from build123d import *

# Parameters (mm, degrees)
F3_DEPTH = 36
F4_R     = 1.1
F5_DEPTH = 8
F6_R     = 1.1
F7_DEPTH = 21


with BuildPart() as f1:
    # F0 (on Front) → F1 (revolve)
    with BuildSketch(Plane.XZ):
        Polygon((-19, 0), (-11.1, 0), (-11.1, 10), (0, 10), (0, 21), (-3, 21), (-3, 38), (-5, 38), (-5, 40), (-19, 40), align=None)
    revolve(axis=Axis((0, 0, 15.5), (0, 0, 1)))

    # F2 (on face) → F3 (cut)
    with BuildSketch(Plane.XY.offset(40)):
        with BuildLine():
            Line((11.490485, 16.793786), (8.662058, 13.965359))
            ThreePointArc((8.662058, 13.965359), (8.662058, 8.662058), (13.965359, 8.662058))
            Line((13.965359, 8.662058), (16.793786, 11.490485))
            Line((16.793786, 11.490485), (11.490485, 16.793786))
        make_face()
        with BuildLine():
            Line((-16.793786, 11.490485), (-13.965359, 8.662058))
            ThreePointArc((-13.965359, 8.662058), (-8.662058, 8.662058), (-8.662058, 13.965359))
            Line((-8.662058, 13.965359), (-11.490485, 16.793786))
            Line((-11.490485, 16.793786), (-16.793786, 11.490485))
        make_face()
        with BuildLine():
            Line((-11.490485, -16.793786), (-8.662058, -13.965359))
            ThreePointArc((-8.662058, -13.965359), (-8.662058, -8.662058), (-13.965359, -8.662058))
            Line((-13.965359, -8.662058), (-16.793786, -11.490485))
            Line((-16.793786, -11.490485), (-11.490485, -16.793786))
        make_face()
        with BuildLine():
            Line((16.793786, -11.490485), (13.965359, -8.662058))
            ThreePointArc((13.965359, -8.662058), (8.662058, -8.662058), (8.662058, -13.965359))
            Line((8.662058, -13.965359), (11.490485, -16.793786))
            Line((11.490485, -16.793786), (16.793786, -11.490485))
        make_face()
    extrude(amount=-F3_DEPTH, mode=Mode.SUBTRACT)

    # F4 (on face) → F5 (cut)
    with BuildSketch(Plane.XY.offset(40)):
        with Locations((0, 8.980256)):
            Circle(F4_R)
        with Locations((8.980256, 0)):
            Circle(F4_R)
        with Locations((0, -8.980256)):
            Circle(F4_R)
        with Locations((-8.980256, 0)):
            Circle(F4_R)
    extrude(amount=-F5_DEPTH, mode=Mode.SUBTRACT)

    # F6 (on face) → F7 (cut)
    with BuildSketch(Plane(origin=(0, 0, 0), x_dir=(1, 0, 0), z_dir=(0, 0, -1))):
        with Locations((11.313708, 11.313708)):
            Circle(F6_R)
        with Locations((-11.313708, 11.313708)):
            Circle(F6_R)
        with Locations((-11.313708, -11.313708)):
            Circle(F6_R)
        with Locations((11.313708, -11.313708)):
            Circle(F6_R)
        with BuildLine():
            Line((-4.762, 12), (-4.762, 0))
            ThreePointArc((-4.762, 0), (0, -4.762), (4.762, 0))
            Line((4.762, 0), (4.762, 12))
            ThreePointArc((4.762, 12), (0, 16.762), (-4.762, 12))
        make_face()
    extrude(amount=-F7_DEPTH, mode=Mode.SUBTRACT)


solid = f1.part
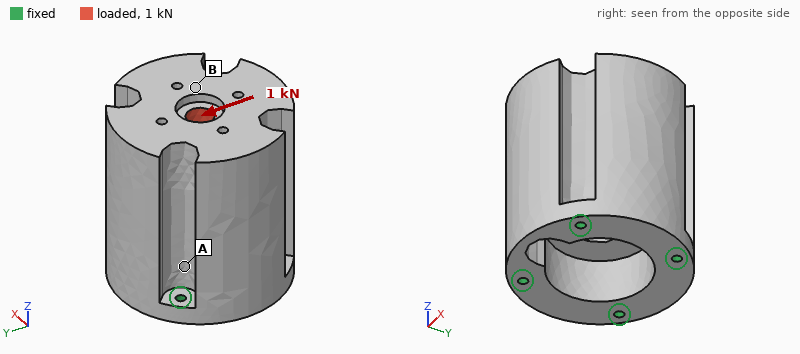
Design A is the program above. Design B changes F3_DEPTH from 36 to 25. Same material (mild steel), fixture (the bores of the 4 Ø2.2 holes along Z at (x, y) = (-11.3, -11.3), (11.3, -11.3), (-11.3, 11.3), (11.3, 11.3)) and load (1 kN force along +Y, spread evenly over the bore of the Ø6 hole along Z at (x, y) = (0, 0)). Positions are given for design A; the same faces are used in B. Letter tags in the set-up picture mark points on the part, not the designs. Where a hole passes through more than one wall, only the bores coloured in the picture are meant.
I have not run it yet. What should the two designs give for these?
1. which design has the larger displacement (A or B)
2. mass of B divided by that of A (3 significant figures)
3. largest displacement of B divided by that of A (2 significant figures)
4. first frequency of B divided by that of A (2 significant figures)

A
1.06
0.20
2.4
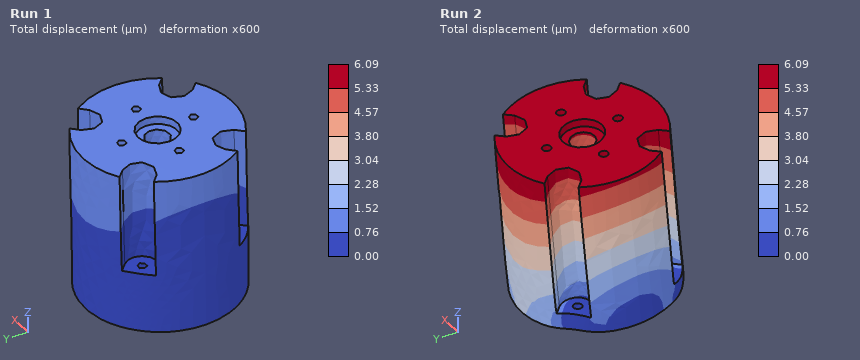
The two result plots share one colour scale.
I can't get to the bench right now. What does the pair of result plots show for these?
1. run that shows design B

Run 1
